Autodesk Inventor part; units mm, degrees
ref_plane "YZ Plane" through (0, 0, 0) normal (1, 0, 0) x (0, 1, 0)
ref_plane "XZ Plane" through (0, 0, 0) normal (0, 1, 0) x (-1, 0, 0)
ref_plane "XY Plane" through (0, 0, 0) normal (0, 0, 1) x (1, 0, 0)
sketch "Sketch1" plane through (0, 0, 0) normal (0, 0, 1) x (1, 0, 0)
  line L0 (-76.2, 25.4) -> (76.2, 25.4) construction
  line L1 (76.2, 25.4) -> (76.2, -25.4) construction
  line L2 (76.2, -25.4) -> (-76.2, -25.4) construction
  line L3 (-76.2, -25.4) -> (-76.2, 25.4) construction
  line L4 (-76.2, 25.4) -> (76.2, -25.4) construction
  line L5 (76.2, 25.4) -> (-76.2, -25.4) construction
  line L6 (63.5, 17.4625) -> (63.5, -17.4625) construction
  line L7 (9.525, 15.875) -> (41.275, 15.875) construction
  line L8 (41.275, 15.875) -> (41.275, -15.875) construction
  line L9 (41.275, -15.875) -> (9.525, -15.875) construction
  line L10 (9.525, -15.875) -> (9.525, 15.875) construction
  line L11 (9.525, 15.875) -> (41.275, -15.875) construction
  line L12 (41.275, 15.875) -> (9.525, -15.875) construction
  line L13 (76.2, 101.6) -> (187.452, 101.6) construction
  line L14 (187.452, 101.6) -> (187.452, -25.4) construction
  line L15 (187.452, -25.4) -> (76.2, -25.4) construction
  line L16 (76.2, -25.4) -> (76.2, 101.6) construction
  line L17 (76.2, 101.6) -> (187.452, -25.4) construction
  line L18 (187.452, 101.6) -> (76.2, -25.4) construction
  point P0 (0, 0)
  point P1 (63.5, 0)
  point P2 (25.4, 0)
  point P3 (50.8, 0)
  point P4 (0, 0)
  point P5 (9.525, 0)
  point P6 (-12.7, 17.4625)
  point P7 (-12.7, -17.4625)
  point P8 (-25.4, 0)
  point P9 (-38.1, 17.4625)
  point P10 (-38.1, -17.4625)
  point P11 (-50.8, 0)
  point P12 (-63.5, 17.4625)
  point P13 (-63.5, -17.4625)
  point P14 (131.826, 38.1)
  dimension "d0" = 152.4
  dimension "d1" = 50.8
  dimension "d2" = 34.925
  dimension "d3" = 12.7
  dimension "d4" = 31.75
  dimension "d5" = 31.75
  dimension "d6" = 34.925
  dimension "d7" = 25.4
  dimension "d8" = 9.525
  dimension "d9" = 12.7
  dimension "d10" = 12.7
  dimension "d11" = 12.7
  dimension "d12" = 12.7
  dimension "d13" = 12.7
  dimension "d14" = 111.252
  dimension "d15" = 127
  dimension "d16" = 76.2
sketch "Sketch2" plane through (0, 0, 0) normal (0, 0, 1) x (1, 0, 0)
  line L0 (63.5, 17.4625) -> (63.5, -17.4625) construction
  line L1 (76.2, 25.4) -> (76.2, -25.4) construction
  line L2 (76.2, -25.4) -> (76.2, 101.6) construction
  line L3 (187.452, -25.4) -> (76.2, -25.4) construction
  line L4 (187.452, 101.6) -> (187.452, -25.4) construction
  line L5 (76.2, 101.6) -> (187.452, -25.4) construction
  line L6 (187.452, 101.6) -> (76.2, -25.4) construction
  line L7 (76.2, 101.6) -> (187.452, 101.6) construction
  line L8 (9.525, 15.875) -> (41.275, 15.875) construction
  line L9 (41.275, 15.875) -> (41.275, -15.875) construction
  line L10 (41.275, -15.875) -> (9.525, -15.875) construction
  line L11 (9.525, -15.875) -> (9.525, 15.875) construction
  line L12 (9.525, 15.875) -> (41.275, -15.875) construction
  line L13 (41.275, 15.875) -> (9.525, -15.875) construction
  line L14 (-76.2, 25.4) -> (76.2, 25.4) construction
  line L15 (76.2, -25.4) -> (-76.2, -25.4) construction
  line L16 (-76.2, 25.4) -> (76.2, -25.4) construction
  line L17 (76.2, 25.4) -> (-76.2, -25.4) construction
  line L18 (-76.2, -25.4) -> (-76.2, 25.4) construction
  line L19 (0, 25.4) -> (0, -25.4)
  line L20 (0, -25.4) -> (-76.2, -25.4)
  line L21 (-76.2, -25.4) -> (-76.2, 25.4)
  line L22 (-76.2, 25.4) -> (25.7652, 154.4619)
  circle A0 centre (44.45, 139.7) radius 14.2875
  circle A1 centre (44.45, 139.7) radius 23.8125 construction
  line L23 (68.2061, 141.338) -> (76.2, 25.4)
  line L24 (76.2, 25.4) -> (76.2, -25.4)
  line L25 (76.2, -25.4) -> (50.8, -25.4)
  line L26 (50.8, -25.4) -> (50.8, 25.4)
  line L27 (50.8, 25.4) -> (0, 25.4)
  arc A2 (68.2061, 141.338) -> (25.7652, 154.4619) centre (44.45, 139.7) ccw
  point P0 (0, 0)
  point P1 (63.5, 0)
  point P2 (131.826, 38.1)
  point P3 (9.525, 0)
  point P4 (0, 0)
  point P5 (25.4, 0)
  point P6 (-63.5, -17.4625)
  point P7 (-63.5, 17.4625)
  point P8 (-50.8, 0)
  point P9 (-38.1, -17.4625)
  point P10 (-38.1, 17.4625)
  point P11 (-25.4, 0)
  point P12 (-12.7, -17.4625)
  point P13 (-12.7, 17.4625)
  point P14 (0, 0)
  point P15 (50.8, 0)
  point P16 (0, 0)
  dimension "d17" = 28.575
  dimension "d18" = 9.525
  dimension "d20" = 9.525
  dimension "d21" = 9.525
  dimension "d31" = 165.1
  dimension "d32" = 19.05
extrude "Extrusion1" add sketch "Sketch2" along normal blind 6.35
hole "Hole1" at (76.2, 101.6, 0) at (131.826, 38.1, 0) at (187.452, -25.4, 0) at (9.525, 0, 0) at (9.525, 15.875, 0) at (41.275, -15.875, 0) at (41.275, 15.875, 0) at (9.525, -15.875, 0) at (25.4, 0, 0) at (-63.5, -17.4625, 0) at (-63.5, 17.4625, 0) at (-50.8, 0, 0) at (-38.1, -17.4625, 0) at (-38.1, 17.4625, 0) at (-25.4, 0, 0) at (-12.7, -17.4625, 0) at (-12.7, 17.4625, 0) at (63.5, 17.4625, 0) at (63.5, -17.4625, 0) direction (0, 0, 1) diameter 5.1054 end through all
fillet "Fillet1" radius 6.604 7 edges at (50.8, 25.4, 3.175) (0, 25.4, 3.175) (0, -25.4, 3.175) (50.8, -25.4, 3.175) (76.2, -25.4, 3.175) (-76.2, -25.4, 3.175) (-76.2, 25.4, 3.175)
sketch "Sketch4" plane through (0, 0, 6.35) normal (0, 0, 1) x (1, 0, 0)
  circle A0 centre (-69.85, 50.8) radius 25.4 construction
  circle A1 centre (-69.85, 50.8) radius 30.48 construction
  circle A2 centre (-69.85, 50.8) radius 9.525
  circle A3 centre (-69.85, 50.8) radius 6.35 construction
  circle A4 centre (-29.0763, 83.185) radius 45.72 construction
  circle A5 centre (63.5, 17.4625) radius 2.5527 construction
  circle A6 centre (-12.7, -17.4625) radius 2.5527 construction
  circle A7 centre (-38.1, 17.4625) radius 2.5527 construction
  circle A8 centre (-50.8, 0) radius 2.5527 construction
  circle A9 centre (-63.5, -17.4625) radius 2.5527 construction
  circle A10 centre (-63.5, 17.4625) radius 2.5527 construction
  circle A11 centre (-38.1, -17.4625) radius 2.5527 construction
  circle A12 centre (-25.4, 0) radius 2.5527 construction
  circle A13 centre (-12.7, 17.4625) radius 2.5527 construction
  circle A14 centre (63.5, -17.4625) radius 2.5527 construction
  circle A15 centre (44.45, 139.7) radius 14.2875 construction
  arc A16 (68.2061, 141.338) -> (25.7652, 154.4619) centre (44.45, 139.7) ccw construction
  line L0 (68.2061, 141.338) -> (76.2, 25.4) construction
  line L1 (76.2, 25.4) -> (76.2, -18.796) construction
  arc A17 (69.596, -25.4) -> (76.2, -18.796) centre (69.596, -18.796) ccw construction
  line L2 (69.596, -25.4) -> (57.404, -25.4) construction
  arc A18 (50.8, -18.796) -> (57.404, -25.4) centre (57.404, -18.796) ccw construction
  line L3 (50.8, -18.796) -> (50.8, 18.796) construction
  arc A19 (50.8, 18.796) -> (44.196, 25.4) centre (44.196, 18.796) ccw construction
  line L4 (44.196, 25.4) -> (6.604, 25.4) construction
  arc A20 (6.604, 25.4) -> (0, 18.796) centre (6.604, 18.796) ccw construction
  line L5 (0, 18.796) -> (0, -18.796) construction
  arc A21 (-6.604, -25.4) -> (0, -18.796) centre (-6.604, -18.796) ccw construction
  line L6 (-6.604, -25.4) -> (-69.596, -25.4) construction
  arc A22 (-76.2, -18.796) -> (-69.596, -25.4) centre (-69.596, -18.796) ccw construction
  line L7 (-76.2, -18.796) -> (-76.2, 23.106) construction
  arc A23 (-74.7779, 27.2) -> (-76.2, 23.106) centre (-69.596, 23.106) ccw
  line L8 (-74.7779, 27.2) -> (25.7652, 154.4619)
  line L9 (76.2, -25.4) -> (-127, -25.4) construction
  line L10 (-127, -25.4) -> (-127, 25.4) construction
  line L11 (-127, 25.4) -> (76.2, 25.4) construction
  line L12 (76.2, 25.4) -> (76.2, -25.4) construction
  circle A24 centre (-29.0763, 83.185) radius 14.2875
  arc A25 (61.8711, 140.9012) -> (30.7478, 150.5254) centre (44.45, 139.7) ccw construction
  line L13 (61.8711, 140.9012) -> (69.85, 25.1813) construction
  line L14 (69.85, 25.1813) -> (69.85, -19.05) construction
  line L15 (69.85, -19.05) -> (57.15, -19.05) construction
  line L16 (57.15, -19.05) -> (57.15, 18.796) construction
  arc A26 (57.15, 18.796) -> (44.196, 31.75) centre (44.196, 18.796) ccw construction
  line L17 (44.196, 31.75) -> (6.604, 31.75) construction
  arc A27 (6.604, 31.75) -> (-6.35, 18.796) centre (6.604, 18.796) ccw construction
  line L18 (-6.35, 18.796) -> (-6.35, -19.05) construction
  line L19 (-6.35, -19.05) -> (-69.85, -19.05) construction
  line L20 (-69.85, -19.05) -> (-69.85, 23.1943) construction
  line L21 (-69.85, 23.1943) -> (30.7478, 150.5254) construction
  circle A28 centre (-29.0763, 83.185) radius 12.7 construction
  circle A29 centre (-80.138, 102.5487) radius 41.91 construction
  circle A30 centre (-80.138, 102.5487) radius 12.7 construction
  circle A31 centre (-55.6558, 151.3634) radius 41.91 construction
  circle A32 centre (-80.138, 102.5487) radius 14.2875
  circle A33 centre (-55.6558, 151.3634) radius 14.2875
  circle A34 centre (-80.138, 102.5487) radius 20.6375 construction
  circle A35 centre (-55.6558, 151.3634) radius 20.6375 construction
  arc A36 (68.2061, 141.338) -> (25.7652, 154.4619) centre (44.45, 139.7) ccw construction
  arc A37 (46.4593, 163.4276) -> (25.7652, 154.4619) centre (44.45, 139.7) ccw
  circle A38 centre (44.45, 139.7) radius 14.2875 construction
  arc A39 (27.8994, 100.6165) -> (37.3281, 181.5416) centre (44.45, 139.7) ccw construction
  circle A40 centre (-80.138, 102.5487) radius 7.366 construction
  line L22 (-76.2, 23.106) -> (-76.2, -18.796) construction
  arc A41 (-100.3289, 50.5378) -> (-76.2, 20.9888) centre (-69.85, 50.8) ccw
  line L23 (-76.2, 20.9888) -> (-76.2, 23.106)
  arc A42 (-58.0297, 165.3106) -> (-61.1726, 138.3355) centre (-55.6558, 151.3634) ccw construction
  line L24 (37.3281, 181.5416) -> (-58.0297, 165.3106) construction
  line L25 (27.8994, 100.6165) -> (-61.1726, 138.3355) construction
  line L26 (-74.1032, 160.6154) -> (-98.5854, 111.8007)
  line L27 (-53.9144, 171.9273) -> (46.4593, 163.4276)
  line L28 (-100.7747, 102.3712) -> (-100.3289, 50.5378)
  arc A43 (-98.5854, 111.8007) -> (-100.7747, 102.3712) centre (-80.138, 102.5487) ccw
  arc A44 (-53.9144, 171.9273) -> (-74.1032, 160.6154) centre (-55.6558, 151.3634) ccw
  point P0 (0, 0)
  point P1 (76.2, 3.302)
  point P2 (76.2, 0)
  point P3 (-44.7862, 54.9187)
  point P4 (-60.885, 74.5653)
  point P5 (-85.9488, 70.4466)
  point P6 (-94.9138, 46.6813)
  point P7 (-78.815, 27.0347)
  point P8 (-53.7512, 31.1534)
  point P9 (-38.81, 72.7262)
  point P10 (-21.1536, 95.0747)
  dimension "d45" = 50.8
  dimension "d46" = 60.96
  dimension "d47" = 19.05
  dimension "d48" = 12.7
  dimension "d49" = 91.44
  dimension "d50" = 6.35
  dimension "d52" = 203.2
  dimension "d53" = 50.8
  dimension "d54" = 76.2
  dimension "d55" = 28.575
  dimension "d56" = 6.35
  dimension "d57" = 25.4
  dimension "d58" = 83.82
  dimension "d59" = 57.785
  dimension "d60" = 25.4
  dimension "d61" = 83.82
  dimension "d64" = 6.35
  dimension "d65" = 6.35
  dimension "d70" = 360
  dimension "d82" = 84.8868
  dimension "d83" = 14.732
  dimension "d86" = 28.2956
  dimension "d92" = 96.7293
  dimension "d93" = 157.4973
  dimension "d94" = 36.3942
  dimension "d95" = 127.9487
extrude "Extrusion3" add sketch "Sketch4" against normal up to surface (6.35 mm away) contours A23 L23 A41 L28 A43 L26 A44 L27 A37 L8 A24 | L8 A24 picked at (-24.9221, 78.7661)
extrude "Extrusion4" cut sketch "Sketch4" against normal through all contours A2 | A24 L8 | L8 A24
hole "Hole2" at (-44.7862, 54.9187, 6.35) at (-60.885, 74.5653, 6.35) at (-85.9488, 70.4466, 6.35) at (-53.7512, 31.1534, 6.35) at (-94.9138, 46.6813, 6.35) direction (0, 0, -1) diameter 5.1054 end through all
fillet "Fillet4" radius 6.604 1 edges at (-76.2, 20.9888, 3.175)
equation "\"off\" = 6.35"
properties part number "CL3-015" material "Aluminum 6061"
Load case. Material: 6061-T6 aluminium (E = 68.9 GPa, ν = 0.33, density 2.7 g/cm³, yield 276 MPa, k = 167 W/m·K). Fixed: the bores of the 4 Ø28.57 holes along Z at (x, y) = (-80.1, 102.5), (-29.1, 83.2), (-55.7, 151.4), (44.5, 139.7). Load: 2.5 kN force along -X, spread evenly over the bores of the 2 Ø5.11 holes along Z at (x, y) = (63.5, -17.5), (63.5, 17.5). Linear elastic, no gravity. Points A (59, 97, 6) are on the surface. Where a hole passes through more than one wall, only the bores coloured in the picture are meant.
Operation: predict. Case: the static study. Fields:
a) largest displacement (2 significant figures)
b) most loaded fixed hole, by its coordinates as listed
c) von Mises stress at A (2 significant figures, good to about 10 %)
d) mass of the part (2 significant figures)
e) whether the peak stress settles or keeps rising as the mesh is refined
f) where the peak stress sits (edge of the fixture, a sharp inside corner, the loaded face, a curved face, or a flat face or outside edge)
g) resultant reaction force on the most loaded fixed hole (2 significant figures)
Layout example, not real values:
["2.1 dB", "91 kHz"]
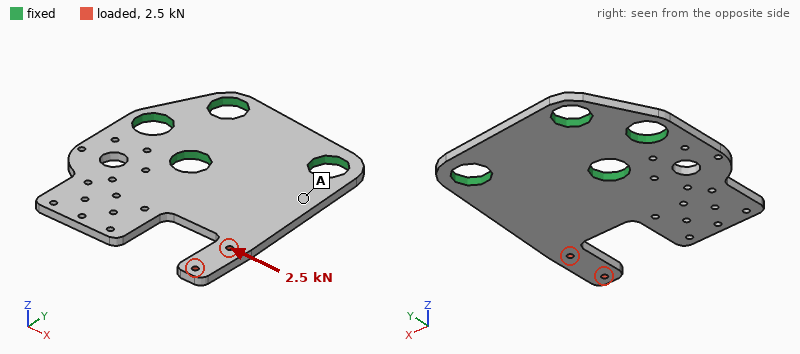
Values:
["0.23 mm", "(-29.1, 83.2)", "10 MPa", "430 g", "keeps rising", "a sharp inside corner", "2.9 kN"]
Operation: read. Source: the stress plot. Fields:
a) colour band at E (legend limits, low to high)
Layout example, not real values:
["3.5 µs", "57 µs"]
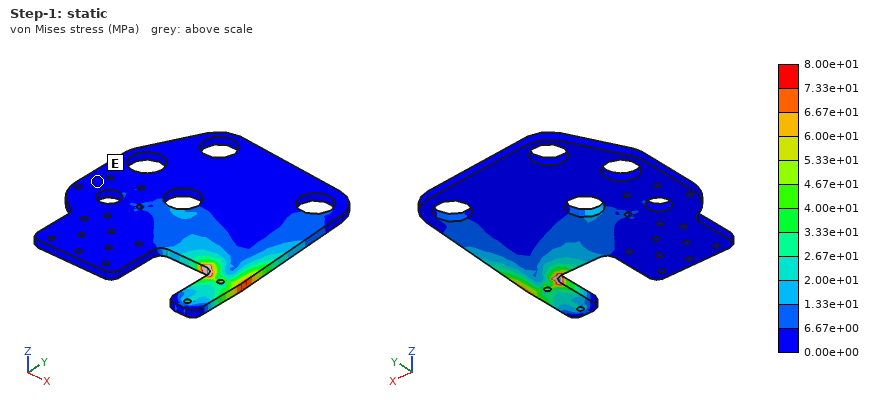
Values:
["0.00e+00 to 6.67e+00 MPa"]
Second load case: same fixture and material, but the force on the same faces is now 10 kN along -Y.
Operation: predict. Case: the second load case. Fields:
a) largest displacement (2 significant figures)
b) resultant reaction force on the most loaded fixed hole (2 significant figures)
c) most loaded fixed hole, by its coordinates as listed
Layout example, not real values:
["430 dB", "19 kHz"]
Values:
["0.17 mm", "9.3 kN", "(44.5, 139.7)"]
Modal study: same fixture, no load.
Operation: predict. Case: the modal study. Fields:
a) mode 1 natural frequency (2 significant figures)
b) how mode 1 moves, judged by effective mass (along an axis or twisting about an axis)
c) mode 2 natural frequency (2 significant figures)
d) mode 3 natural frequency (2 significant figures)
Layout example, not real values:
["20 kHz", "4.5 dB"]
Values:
["500 Hz", "along Z", "640 Hz", "1500 Hz"]
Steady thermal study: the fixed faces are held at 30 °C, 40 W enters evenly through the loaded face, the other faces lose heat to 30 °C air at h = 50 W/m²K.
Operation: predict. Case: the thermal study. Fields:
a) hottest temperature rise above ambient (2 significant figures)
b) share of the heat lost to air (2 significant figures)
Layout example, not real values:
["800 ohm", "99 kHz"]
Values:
["70 K", "47 %"]
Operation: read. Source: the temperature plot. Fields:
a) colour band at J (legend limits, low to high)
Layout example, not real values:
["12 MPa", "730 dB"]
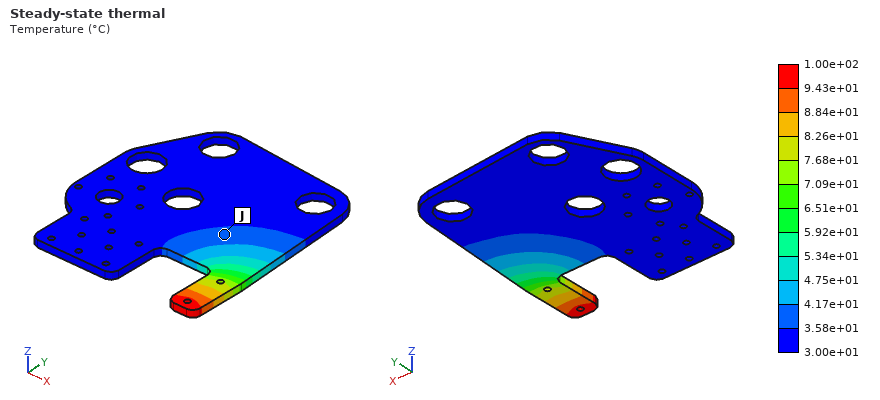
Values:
["3.58e+01 to 4.17e+01 °C"]
